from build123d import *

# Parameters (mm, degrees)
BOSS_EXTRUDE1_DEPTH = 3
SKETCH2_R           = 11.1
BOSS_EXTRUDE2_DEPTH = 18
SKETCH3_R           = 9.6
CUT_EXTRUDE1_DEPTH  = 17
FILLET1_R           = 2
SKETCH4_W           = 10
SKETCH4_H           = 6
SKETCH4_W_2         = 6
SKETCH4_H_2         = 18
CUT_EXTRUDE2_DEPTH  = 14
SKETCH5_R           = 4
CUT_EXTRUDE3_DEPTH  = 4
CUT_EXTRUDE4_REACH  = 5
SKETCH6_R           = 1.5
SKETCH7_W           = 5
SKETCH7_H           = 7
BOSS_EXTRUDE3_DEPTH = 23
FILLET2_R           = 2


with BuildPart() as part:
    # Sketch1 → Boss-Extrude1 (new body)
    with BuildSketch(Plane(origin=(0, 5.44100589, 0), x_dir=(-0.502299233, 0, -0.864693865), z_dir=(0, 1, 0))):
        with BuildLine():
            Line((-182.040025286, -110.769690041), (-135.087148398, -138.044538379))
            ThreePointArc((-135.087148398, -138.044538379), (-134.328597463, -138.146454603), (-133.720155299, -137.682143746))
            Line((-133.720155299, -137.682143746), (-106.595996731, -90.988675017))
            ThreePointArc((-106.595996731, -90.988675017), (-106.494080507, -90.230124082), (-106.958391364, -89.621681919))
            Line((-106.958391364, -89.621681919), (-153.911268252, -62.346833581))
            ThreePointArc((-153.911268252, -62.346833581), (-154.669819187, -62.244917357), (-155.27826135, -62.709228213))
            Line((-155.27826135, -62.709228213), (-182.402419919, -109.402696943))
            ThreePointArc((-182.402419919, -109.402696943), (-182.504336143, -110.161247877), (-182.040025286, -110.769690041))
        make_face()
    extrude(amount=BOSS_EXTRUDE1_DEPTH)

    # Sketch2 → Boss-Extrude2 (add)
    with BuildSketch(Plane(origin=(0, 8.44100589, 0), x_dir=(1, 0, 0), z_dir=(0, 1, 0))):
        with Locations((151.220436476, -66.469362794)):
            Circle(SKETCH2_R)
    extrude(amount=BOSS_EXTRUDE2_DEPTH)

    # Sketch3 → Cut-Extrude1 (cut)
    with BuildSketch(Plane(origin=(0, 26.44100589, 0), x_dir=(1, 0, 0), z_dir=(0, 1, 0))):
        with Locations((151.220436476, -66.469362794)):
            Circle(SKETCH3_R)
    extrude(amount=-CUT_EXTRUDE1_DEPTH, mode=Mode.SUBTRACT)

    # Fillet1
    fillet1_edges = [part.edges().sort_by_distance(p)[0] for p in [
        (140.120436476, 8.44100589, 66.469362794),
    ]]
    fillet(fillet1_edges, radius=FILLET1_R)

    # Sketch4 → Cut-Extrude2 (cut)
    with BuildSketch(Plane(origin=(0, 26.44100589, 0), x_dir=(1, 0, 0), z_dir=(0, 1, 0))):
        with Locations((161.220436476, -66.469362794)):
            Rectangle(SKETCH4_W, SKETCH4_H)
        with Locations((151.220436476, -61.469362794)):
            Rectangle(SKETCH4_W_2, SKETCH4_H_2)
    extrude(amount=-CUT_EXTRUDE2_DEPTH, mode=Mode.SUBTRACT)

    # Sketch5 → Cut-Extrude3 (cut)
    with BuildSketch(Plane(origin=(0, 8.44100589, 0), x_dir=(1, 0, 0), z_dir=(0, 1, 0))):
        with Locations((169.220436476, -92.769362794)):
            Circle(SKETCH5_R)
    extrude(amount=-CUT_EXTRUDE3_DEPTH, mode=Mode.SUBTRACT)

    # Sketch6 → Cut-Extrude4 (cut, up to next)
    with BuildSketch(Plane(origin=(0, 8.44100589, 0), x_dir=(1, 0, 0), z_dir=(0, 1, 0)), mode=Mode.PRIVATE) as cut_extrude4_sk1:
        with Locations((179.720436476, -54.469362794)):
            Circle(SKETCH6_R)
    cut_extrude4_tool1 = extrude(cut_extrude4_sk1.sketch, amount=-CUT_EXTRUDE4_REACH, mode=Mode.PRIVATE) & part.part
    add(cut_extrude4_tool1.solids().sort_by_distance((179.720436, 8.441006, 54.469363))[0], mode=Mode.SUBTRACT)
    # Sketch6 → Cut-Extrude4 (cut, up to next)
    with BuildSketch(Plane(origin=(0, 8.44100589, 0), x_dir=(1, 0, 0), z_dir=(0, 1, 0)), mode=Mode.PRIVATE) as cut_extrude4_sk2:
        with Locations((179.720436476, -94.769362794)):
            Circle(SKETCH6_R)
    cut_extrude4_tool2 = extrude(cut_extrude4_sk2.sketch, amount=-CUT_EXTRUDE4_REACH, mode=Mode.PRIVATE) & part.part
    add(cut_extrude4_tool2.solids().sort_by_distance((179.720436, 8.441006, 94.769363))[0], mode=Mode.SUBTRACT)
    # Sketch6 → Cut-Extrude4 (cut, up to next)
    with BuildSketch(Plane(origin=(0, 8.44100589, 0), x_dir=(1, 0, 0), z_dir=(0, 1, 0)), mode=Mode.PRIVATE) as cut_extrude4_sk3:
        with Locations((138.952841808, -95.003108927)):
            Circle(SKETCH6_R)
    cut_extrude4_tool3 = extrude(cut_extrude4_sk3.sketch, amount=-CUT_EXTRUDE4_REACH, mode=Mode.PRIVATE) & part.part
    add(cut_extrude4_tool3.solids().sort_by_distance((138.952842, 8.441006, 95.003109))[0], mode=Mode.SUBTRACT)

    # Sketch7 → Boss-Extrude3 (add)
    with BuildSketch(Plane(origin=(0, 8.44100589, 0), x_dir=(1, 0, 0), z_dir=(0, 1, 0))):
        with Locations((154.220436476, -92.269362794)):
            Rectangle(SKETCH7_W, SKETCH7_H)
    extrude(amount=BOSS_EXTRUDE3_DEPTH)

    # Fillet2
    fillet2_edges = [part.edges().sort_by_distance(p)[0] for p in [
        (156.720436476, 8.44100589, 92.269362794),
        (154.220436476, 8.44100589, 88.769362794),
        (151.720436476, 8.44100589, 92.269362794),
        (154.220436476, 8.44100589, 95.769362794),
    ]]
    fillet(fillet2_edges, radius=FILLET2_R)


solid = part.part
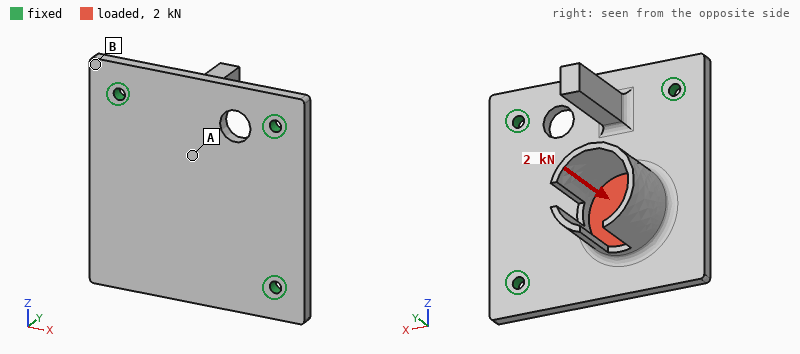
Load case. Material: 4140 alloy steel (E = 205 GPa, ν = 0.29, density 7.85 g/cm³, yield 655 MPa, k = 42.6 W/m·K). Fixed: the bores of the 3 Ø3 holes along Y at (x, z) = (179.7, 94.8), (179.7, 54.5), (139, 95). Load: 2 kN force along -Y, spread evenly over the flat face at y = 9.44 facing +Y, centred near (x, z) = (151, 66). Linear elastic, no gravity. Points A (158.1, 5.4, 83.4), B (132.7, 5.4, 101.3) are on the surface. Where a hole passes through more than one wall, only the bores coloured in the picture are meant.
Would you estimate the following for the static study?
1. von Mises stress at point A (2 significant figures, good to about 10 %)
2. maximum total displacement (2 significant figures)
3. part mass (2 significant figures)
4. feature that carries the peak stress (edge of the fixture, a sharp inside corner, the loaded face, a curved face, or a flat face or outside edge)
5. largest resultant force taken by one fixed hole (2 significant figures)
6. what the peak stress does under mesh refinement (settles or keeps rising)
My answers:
130 MPa
0.47 mm
94 g
edge of the fixture
1.2 kN
keeps rising
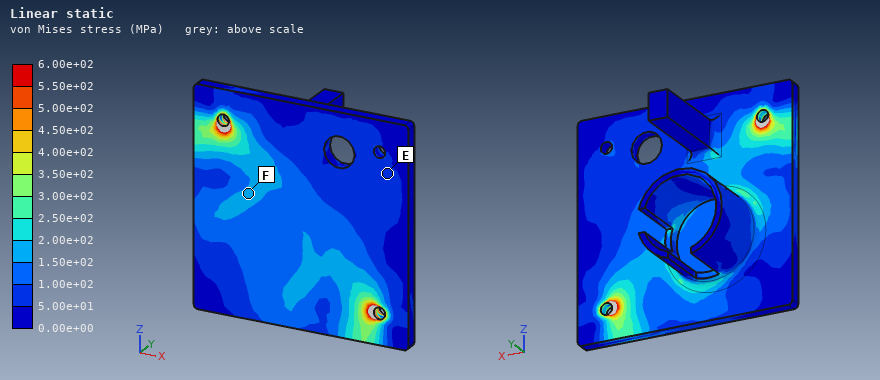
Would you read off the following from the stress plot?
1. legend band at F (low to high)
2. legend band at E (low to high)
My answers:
1.50e+02 to 2.00e+02 MPa
5.00e+01 to 1.00e+02 MPa
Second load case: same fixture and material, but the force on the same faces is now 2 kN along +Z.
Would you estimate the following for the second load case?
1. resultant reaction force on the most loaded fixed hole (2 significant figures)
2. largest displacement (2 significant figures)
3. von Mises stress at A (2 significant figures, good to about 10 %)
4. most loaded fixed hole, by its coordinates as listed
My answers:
1.1 kN
60 µm
16 MPa
(139, 95)
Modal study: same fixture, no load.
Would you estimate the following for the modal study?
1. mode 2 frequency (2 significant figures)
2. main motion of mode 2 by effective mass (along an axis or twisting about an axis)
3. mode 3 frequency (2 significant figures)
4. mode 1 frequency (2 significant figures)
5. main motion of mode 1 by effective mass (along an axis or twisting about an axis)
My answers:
4900 Hz
along Y
5400 Hz
1900 Hz
along Y
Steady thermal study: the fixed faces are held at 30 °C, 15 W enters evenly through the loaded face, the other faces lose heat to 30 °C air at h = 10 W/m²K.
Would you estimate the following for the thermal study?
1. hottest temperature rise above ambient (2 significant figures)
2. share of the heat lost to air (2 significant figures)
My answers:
53 K
16 %
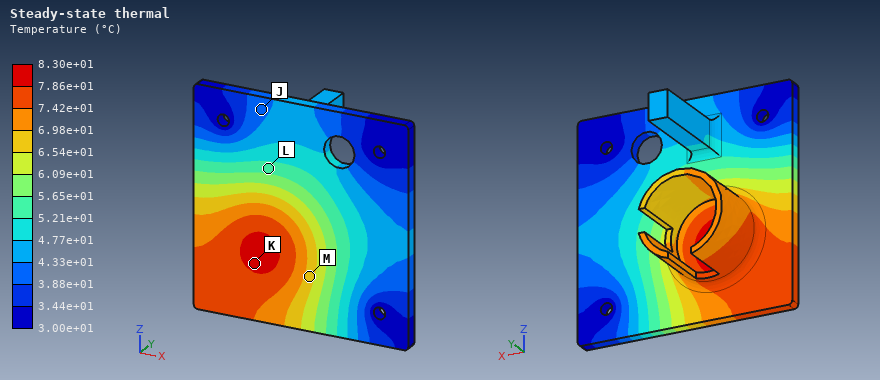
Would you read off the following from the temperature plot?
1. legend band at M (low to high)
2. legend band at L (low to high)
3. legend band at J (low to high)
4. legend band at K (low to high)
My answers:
6.54e+01 to 6.98e+01 °C
5.21e+01 to 5.65e+01 °C
3.88e+01 to 4.33e+01 °C
7.86e+01 to 8.30e+01 °C
